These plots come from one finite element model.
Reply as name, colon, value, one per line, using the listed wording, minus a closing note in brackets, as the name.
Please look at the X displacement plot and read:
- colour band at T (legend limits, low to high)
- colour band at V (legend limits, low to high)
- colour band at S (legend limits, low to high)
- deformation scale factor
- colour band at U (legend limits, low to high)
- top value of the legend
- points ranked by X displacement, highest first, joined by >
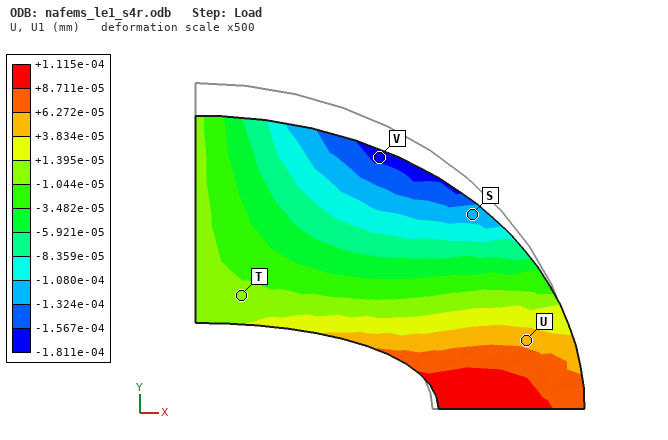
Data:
colour band at T: -1.044e-05 to +1.395e-05 mm
colour band at V: -1.811e-04 to -1.567e-04 mm
colour band at S: -1.324e-04 to -1.080e-04 mm
deformation scale factor: 500
colour band at U: +3.834e-05 to +6.272e-05 mm
top value of the legend: +1.115e-04 mm
points ranked by X displacement, highest first, joined by >: U > T > S > V
